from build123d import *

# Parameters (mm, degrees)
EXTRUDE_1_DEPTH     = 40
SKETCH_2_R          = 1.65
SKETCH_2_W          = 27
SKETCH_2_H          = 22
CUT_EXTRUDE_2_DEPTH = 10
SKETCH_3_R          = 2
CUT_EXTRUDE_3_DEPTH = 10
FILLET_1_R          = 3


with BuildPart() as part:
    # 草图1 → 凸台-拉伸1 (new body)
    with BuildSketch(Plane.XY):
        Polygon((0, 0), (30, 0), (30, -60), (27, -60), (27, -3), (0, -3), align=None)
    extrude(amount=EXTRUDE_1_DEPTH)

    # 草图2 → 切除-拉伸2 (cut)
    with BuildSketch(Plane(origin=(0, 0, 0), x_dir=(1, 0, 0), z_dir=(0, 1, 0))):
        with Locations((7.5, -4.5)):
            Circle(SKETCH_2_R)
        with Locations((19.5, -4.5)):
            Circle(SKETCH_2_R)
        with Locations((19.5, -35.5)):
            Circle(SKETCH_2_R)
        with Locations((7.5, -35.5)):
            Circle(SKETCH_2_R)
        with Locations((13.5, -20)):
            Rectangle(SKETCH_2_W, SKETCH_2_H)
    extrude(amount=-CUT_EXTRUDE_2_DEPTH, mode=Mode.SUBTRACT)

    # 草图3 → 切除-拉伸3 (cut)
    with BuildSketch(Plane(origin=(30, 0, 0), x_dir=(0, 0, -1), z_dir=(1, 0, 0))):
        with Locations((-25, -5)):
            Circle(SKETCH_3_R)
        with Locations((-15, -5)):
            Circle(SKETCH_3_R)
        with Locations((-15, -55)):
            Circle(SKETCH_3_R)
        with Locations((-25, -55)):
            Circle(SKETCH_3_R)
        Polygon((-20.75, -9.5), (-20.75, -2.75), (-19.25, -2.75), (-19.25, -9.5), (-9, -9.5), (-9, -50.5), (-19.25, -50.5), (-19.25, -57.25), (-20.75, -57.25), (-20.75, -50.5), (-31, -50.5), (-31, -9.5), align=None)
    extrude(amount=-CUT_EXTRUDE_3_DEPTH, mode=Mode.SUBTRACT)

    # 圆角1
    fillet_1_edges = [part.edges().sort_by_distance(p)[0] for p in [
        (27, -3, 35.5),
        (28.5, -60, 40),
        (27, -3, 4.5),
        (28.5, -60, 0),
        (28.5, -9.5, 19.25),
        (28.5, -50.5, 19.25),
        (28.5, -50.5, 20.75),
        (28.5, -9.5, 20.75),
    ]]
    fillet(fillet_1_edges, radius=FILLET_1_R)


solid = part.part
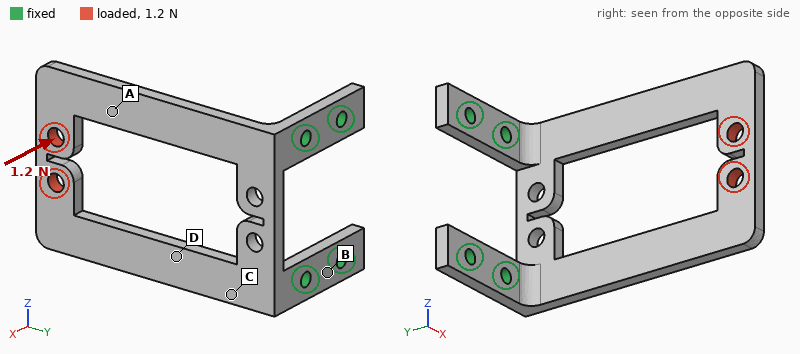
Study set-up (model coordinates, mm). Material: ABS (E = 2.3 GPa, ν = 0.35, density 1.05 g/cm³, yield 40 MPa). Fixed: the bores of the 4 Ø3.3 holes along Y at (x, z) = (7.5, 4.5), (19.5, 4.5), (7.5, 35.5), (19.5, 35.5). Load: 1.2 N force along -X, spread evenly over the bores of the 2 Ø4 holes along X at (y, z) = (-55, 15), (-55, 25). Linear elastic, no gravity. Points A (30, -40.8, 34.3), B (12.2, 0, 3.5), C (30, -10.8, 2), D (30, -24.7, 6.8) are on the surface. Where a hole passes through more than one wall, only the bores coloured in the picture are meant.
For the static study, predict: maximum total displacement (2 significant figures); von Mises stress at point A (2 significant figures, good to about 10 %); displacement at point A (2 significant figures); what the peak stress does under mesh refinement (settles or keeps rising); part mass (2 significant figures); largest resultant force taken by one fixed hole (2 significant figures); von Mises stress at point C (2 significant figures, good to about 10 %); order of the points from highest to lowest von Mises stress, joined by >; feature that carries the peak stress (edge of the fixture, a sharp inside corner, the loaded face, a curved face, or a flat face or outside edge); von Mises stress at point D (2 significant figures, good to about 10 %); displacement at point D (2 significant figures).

0.90 mm
0.65 MPa
0.50 mm
keeps rising
5.9 g
0.60 N
1.9 MPa
C > D > A > B
edge of the fixture
1.4 MPa
0.22 mm
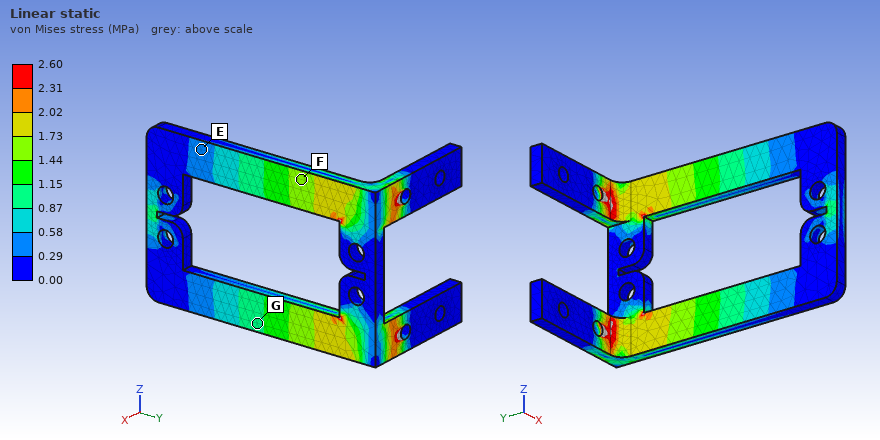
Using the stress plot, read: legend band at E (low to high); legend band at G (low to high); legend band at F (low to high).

0.29 to 0.58 MPa
0.87 to 1.15 MPa
1.44 to 1.73 MPa
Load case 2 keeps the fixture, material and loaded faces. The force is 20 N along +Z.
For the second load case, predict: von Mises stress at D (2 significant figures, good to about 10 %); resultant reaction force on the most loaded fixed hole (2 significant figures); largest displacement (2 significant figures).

1.4 MPa
33 N
0.81 mm
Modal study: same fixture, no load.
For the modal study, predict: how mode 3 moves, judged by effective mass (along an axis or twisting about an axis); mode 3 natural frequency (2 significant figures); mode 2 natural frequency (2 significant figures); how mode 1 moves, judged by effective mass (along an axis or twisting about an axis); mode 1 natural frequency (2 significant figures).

along Z
630 Hz
450 Hz
along X
150 Hz
